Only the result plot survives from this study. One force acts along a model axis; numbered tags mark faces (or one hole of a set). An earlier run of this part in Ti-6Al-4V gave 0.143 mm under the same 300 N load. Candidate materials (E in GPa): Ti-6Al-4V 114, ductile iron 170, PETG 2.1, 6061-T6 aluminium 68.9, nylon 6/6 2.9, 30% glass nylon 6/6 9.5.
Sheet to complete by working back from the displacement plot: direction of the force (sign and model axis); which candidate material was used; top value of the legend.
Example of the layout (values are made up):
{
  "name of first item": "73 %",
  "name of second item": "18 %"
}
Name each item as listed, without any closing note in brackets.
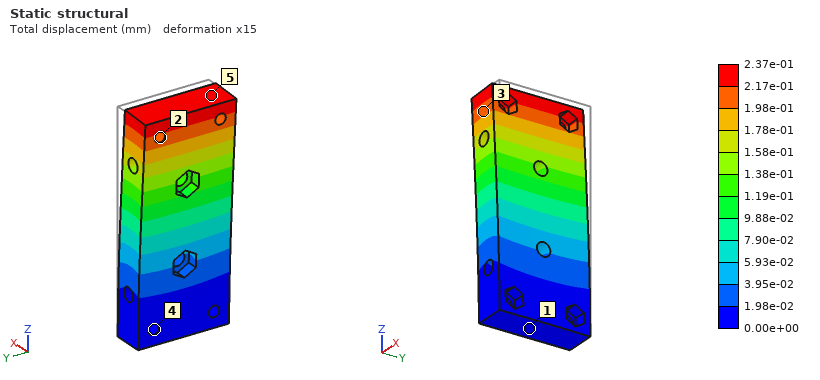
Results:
{
  "direction of the force": "-X",
  "which candidate material was used": "6061-T6 aluminium",
  "top value of the legend": "2.37e-01 mm"
}
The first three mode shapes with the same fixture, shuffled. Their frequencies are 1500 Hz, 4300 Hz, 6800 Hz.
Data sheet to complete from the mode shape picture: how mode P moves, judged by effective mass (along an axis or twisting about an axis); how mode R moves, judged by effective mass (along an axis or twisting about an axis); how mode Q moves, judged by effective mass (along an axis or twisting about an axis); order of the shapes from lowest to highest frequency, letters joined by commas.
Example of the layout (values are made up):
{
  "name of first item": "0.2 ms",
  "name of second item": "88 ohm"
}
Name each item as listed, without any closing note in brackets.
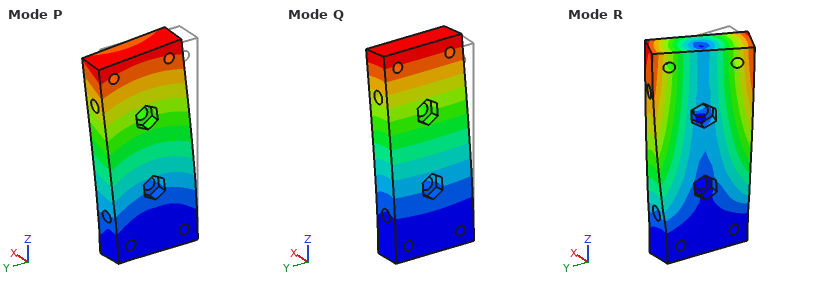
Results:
{
  "how mode P moves, judged by effective mass": "along Y",
  "how mode R moves, judged by effective mass": "twisting about Z",
  "how mode Q moves, judged by effective mass": "along X",
  "order of the shapes from lowest to highest frequency, letters joined by commas": "Q, P, R"
}
